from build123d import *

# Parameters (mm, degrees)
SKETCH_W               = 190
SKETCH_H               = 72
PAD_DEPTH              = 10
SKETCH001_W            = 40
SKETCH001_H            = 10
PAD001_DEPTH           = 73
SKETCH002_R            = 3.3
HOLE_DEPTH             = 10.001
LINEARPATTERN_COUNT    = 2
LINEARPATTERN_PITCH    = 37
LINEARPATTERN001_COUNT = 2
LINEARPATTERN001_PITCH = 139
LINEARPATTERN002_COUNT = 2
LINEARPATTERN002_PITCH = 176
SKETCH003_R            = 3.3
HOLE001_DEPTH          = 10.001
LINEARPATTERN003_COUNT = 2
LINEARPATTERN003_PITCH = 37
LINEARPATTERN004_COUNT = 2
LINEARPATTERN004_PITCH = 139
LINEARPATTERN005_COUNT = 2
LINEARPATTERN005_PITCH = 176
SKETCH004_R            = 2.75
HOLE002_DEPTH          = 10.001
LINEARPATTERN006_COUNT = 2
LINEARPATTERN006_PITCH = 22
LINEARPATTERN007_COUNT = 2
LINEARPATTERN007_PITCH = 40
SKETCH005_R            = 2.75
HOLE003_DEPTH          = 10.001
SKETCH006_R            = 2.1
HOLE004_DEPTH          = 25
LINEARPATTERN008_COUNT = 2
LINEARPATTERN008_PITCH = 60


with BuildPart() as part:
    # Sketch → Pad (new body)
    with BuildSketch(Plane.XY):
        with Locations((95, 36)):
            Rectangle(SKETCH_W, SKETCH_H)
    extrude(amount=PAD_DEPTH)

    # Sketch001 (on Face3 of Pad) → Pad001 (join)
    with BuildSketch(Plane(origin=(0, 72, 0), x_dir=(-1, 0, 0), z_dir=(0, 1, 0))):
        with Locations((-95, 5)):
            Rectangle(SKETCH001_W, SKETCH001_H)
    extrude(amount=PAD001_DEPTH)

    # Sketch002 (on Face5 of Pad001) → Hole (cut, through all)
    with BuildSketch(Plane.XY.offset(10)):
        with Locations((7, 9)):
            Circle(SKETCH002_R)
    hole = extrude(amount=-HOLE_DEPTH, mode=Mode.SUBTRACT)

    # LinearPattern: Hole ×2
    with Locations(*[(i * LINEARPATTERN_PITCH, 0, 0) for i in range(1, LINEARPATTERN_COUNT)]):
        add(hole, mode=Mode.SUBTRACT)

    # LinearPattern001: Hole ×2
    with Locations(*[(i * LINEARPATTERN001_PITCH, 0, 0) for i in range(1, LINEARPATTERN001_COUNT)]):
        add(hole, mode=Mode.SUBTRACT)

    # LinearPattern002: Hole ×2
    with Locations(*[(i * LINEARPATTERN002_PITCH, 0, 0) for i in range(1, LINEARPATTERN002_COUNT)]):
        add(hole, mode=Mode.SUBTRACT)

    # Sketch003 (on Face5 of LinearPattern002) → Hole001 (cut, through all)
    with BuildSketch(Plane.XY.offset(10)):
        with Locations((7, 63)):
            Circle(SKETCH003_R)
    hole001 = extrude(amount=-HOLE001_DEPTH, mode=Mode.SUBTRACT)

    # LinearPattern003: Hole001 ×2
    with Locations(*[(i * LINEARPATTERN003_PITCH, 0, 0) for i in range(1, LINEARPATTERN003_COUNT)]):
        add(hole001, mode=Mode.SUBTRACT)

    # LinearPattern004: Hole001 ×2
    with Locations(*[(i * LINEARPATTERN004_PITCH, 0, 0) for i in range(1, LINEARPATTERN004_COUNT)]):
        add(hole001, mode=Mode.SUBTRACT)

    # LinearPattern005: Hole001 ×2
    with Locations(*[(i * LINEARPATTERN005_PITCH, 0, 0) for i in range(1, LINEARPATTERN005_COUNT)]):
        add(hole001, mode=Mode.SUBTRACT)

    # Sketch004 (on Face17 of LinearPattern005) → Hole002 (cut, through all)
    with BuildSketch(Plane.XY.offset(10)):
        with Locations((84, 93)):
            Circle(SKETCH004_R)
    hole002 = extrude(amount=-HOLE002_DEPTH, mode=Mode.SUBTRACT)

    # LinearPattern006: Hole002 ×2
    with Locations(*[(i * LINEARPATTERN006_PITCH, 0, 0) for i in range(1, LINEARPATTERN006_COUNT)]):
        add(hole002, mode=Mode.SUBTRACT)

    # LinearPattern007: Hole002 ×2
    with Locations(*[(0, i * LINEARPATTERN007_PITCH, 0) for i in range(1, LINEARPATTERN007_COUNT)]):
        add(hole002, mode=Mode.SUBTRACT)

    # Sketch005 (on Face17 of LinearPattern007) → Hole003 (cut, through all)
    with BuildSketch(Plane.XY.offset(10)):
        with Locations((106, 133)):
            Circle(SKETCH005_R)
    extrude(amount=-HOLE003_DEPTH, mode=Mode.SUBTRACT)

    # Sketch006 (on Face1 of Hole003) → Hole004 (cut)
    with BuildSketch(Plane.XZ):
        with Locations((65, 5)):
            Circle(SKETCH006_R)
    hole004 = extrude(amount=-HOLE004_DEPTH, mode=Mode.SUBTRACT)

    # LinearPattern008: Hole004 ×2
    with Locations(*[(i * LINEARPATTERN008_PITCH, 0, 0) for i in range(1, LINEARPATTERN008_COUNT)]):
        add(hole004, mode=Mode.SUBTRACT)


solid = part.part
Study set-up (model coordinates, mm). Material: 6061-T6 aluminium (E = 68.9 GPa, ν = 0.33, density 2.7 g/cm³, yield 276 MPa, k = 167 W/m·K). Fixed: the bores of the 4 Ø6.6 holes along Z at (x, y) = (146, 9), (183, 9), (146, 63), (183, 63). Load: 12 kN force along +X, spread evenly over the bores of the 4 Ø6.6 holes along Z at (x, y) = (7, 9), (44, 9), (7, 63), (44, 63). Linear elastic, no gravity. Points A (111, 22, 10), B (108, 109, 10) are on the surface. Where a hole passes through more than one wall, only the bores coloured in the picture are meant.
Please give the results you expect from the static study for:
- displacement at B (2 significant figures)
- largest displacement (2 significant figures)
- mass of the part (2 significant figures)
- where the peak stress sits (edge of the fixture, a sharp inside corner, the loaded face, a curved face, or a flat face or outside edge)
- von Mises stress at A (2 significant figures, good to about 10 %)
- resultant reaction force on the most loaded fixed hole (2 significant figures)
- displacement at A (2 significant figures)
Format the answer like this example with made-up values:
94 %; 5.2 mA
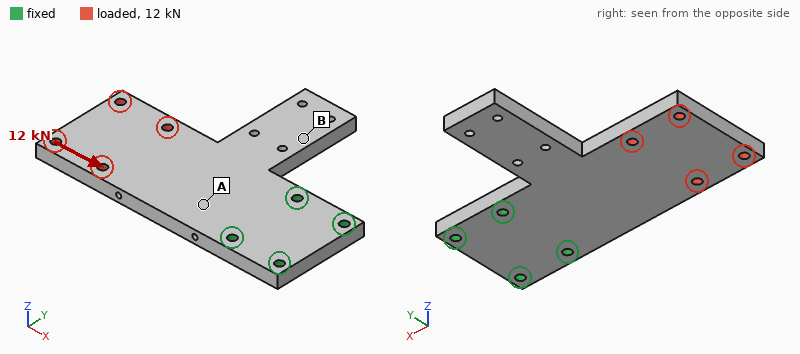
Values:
12 µm; 41 µm; 440 g; a curved face; 16 MPa; 5.1 kN; 11 µm
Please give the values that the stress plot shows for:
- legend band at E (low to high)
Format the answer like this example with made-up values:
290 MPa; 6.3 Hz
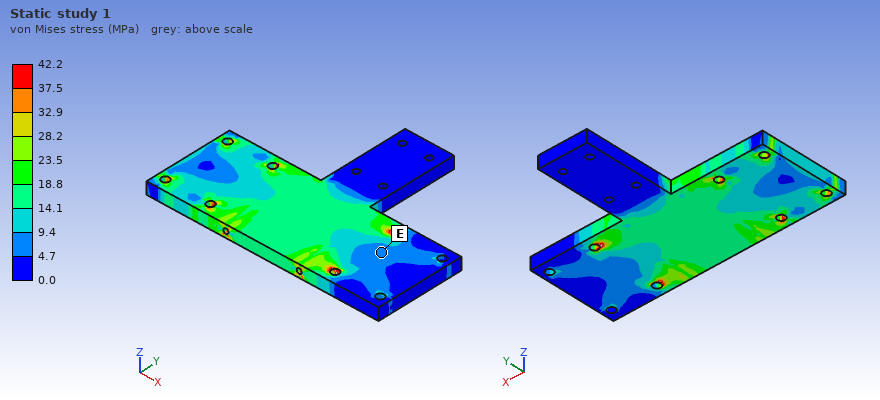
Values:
4.7 to 9.4 MPa
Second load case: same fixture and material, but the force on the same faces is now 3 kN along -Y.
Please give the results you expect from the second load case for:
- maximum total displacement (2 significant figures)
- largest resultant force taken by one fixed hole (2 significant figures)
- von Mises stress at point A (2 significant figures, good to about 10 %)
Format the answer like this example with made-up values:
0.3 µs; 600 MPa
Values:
0.14 mm; 6.2 kN; 15 MPa
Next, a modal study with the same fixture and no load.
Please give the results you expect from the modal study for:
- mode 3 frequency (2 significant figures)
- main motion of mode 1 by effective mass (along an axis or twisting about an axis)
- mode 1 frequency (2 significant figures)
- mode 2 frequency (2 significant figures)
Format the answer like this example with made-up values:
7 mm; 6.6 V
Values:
1900 Hz; along Z; 380 Hz; 740 Hz
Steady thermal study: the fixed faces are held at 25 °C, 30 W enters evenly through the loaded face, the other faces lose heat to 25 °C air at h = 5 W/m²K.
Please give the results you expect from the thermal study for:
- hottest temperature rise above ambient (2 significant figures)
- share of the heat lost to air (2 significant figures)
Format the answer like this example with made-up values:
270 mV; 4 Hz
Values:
31 K; 8.8 %
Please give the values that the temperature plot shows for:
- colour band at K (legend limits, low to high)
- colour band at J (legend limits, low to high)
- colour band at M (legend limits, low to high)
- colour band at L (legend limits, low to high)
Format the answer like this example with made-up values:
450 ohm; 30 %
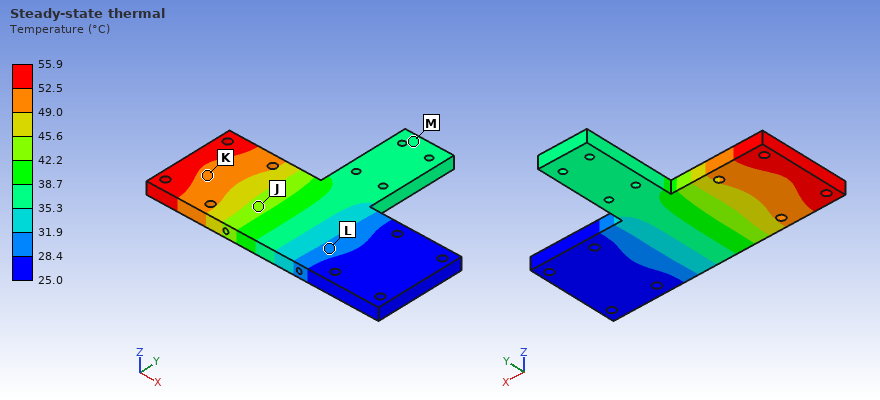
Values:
49.0 to 52.5 °C; 42.2 to 45.6 °C; 35.3 to 38.7 °C; 28.4 to 31.9 °C
